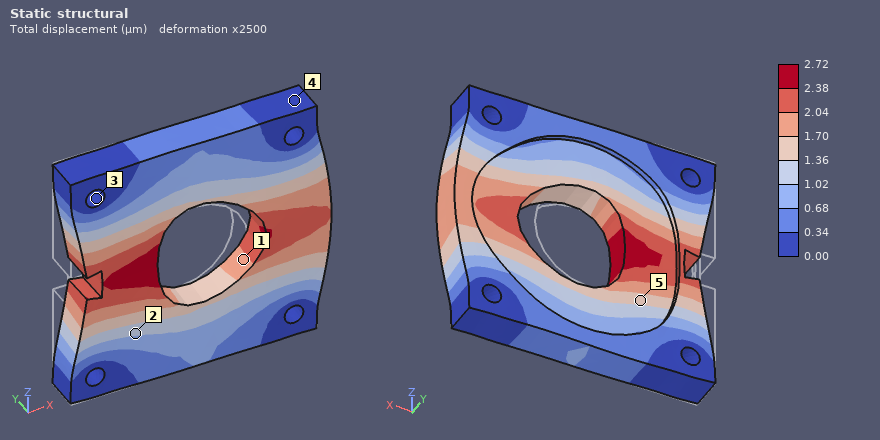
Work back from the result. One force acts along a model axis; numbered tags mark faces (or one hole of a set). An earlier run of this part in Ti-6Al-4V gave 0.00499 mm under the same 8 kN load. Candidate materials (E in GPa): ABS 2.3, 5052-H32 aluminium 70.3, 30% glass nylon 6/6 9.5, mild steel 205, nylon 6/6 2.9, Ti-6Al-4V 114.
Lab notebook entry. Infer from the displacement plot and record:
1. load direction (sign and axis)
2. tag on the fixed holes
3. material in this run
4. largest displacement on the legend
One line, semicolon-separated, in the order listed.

+X; 3; mild steel; 2.72 µm
